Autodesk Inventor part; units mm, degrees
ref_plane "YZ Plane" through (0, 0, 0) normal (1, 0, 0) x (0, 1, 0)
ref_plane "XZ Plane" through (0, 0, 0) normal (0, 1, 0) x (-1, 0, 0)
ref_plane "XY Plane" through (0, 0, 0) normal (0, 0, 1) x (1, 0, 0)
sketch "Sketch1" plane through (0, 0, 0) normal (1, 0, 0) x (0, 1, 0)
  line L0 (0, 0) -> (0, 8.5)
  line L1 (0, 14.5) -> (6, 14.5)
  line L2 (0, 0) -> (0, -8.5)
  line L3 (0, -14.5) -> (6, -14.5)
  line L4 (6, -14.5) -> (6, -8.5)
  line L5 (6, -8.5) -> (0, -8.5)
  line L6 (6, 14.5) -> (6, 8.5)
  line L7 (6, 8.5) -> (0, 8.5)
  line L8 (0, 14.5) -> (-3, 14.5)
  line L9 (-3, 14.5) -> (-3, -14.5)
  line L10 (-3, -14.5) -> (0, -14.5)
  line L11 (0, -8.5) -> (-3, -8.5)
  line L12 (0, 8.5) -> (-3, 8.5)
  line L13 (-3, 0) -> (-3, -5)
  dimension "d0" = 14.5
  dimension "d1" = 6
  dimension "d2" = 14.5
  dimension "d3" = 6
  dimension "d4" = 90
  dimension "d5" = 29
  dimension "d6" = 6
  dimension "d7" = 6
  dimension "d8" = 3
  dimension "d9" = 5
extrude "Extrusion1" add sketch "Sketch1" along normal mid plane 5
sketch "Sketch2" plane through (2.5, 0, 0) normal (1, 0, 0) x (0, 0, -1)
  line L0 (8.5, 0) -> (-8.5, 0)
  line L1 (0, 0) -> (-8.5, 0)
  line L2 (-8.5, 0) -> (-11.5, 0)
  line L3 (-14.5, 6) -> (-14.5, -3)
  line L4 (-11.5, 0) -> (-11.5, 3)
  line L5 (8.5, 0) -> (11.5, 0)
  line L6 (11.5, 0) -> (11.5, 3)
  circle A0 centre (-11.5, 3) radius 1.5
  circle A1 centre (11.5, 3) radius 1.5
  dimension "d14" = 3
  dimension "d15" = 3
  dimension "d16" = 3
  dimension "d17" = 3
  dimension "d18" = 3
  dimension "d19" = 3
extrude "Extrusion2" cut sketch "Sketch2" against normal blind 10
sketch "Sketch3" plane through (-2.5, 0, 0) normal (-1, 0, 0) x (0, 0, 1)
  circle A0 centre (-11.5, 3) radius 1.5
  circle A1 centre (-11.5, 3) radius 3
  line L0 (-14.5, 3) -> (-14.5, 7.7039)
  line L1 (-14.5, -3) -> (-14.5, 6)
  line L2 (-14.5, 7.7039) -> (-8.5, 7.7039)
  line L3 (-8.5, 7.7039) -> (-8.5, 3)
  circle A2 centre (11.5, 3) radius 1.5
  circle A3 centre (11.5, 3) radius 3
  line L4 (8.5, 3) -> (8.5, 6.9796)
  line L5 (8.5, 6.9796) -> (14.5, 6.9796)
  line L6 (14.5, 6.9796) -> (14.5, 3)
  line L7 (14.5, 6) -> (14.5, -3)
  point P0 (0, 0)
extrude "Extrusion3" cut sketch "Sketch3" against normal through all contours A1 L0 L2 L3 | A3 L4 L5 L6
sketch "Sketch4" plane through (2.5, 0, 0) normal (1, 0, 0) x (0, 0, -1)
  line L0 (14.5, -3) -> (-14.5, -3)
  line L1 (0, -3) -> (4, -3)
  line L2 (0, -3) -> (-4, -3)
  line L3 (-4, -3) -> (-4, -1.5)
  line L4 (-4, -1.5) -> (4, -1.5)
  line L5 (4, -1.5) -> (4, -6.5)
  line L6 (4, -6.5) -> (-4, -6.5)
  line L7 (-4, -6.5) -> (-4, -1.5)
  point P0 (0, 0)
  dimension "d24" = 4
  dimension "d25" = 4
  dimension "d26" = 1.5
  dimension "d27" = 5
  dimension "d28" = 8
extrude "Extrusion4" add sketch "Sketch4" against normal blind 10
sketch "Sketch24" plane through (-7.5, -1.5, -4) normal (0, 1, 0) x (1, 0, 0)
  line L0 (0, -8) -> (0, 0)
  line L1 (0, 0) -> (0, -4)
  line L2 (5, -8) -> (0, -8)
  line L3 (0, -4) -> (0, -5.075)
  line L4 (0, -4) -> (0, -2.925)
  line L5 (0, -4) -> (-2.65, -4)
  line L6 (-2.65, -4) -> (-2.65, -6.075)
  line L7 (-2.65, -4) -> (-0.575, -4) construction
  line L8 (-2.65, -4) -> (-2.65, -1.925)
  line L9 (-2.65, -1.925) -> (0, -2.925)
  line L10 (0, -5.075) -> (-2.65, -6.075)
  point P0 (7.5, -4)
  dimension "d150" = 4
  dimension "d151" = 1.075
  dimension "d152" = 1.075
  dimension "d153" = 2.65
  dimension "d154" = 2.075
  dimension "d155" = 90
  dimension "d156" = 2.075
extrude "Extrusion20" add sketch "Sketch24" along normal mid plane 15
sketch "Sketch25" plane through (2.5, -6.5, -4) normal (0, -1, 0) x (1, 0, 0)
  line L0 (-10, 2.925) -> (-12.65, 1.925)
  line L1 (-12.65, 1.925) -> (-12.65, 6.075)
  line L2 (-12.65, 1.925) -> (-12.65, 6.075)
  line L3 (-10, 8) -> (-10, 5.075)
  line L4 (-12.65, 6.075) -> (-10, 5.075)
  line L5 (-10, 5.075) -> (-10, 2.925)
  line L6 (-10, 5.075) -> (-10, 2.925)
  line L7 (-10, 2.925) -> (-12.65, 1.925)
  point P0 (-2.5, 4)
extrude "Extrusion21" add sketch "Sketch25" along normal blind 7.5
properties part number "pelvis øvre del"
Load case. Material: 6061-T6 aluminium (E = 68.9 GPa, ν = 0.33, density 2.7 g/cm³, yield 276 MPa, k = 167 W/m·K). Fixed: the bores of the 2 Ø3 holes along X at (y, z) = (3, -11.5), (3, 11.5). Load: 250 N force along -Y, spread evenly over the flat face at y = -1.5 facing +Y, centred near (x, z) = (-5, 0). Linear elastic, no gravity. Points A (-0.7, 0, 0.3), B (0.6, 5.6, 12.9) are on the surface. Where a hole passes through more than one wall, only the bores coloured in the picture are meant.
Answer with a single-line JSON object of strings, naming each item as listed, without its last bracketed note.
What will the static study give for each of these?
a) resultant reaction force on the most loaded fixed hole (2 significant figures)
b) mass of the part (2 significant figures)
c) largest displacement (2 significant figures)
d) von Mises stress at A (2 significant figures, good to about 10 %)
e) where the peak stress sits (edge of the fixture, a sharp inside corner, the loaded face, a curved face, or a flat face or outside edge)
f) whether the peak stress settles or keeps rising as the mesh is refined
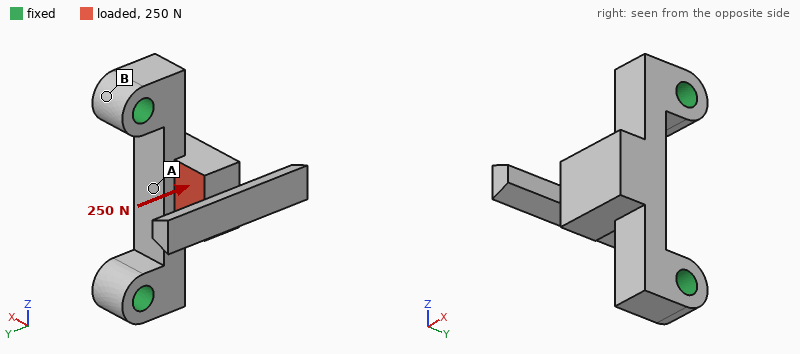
{"resultant reaction force on the most loaded fixed hole": "170 N", "mass of the part": "3.2 g", "largest displacement": "0.10 mm", "von Mises stress at A": "20 MPa", "where the peak stress sits": "a sharp inside corner", "whether the peak stress settles or keeps rising as the mesh is refined": "keeps rising"}
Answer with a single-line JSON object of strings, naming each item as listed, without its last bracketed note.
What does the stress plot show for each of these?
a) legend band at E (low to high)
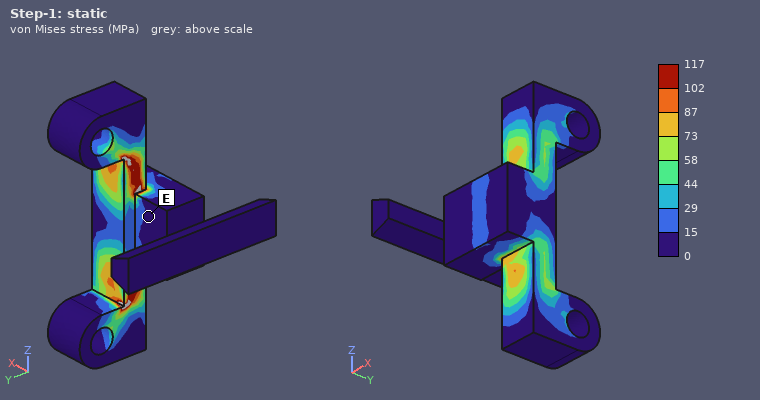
{"legend band at E": "0 to 15 MPa"}
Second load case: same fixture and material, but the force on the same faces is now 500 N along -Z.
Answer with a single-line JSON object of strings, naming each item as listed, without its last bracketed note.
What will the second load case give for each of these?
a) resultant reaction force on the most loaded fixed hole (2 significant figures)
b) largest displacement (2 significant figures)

{"resultant reaction force on the most loaded fixed hole": "290 N", "largest displacement": "32 µm"}
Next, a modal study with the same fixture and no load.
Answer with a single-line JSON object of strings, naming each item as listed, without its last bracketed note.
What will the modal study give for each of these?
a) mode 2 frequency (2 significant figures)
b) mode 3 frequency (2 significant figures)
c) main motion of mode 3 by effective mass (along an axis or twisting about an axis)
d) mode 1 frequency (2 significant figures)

{"mode 2 frequency": "18 kHz", "mode 3 frequency": "19 kHz", "main motion of mode 3 by effective mass": "along X", "mode 1 frequency": "7600 Hz"}
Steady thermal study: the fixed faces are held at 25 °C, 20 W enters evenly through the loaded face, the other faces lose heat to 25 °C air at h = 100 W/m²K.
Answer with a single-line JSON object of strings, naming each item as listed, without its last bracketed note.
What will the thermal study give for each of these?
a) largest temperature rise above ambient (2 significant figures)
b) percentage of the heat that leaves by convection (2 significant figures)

{"largest temperature rise above ambient": "47 K", "percentage of the heat that leaves by convection": "12 %"}
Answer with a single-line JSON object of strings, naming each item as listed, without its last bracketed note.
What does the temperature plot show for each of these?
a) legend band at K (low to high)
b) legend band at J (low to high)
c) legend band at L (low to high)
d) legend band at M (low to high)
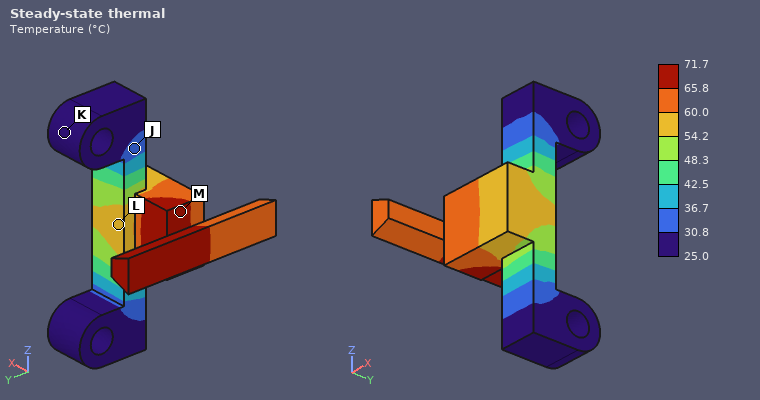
{"legend band at K": "25.0 to 30.8 °C", "legend band at J": "30.8 to 36.7 °C", "legend band at L": "54.2 to 60.0 °C", "legend band at M": "65.8 to 71.7 °C"}
